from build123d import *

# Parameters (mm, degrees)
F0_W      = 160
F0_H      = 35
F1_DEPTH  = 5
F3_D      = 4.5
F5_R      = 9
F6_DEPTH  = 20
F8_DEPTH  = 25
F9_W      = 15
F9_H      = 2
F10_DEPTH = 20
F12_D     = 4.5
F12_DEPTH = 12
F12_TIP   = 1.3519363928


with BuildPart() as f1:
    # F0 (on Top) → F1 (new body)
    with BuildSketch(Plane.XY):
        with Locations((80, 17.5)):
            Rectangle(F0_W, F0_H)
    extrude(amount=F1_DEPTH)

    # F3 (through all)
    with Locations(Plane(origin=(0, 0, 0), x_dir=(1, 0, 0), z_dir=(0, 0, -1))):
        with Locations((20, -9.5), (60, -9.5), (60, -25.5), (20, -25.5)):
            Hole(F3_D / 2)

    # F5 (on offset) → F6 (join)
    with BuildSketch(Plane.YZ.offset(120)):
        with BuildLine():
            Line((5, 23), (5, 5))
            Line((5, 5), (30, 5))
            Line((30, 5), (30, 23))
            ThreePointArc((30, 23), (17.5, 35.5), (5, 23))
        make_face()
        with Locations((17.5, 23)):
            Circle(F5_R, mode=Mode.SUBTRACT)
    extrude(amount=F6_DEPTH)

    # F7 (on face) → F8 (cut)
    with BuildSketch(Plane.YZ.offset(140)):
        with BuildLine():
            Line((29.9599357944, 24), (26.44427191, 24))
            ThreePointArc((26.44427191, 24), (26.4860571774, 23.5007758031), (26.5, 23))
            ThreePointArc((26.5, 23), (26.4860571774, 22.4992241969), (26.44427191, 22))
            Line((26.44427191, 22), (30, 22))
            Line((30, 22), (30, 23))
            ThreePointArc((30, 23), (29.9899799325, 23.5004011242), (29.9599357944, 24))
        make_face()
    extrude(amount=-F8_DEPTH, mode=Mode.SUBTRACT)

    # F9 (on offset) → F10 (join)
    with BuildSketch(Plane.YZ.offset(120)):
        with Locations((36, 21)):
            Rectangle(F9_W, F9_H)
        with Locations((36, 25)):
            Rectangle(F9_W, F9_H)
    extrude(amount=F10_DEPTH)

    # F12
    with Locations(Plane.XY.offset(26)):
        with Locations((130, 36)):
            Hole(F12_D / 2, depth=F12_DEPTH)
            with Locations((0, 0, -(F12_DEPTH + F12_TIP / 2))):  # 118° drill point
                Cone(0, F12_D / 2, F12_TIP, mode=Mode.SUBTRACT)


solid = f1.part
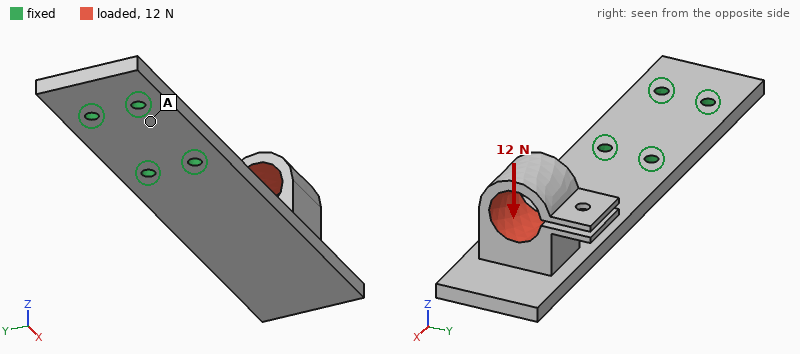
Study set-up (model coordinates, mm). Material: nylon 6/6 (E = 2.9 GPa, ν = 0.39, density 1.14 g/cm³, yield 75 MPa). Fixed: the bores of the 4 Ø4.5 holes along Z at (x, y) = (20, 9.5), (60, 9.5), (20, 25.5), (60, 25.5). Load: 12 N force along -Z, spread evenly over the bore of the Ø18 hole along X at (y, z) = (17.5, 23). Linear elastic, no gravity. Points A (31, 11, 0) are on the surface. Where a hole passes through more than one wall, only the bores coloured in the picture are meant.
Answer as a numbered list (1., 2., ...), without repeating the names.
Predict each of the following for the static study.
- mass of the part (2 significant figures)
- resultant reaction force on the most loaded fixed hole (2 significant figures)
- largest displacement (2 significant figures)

1. 43 g
2. 7.1 N
3. 2.0 mm
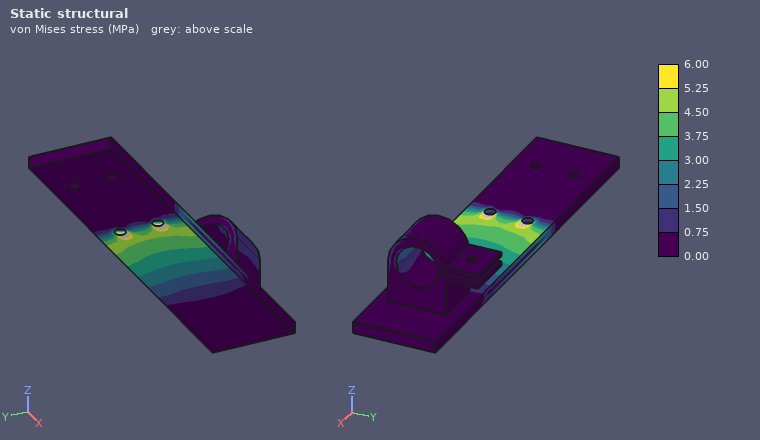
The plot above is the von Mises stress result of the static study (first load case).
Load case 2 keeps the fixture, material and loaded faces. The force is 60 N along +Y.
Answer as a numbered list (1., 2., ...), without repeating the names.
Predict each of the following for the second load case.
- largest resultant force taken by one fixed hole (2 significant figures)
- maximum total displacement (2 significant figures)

1. 180 N
2. 1.8 mm
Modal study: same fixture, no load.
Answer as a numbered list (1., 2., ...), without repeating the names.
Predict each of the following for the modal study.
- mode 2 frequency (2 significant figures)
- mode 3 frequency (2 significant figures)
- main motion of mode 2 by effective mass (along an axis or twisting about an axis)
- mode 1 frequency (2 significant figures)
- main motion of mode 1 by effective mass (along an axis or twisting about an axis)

1. 340 Hz
2. 560 Hz
3. along Y
4. 96 Hz
5. along Z
